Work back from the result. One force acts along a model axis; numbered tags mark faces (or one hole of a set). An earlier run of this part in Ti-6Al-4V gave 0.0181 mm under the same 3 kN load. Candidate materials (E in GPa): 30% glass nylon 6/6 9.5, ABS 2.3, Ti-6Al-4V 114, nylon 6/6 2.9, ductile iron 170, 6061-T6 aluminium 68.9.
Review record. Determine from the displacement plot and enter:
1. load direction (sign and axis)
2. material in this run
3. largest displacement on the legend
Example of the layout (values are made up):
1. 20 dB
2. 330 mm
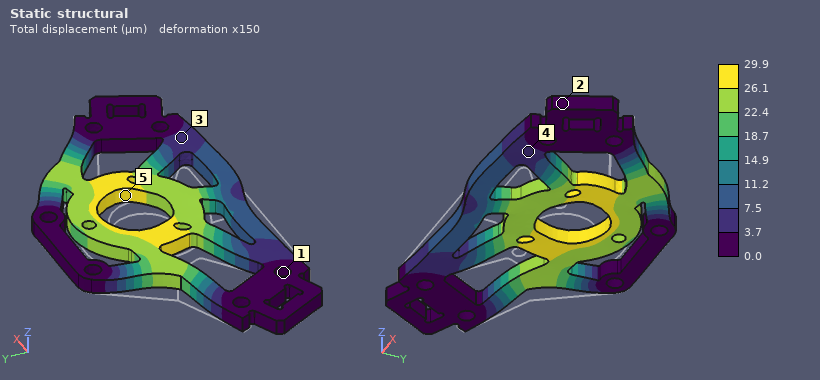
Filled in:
1. +X
2. 6061-T6 aluminium
3. 29.9 µm
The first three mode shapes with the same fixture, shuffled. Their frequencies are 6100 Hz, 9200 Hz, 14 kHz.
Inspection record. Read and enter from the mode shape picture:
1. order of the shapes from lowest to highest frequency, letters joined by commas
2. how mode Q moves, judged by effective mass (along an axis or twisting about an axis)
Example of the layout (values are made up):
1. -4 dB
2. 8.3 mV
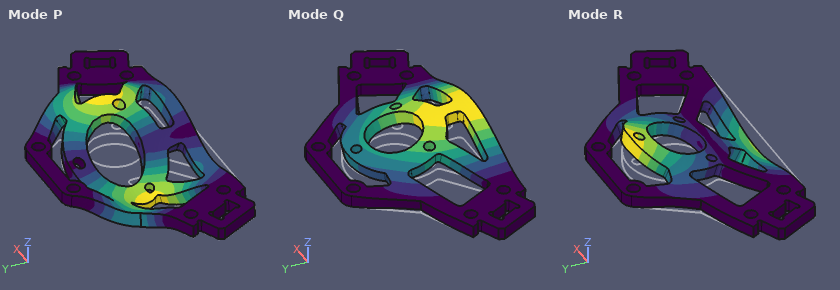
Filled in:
1. Q, R, P
2. along Z
